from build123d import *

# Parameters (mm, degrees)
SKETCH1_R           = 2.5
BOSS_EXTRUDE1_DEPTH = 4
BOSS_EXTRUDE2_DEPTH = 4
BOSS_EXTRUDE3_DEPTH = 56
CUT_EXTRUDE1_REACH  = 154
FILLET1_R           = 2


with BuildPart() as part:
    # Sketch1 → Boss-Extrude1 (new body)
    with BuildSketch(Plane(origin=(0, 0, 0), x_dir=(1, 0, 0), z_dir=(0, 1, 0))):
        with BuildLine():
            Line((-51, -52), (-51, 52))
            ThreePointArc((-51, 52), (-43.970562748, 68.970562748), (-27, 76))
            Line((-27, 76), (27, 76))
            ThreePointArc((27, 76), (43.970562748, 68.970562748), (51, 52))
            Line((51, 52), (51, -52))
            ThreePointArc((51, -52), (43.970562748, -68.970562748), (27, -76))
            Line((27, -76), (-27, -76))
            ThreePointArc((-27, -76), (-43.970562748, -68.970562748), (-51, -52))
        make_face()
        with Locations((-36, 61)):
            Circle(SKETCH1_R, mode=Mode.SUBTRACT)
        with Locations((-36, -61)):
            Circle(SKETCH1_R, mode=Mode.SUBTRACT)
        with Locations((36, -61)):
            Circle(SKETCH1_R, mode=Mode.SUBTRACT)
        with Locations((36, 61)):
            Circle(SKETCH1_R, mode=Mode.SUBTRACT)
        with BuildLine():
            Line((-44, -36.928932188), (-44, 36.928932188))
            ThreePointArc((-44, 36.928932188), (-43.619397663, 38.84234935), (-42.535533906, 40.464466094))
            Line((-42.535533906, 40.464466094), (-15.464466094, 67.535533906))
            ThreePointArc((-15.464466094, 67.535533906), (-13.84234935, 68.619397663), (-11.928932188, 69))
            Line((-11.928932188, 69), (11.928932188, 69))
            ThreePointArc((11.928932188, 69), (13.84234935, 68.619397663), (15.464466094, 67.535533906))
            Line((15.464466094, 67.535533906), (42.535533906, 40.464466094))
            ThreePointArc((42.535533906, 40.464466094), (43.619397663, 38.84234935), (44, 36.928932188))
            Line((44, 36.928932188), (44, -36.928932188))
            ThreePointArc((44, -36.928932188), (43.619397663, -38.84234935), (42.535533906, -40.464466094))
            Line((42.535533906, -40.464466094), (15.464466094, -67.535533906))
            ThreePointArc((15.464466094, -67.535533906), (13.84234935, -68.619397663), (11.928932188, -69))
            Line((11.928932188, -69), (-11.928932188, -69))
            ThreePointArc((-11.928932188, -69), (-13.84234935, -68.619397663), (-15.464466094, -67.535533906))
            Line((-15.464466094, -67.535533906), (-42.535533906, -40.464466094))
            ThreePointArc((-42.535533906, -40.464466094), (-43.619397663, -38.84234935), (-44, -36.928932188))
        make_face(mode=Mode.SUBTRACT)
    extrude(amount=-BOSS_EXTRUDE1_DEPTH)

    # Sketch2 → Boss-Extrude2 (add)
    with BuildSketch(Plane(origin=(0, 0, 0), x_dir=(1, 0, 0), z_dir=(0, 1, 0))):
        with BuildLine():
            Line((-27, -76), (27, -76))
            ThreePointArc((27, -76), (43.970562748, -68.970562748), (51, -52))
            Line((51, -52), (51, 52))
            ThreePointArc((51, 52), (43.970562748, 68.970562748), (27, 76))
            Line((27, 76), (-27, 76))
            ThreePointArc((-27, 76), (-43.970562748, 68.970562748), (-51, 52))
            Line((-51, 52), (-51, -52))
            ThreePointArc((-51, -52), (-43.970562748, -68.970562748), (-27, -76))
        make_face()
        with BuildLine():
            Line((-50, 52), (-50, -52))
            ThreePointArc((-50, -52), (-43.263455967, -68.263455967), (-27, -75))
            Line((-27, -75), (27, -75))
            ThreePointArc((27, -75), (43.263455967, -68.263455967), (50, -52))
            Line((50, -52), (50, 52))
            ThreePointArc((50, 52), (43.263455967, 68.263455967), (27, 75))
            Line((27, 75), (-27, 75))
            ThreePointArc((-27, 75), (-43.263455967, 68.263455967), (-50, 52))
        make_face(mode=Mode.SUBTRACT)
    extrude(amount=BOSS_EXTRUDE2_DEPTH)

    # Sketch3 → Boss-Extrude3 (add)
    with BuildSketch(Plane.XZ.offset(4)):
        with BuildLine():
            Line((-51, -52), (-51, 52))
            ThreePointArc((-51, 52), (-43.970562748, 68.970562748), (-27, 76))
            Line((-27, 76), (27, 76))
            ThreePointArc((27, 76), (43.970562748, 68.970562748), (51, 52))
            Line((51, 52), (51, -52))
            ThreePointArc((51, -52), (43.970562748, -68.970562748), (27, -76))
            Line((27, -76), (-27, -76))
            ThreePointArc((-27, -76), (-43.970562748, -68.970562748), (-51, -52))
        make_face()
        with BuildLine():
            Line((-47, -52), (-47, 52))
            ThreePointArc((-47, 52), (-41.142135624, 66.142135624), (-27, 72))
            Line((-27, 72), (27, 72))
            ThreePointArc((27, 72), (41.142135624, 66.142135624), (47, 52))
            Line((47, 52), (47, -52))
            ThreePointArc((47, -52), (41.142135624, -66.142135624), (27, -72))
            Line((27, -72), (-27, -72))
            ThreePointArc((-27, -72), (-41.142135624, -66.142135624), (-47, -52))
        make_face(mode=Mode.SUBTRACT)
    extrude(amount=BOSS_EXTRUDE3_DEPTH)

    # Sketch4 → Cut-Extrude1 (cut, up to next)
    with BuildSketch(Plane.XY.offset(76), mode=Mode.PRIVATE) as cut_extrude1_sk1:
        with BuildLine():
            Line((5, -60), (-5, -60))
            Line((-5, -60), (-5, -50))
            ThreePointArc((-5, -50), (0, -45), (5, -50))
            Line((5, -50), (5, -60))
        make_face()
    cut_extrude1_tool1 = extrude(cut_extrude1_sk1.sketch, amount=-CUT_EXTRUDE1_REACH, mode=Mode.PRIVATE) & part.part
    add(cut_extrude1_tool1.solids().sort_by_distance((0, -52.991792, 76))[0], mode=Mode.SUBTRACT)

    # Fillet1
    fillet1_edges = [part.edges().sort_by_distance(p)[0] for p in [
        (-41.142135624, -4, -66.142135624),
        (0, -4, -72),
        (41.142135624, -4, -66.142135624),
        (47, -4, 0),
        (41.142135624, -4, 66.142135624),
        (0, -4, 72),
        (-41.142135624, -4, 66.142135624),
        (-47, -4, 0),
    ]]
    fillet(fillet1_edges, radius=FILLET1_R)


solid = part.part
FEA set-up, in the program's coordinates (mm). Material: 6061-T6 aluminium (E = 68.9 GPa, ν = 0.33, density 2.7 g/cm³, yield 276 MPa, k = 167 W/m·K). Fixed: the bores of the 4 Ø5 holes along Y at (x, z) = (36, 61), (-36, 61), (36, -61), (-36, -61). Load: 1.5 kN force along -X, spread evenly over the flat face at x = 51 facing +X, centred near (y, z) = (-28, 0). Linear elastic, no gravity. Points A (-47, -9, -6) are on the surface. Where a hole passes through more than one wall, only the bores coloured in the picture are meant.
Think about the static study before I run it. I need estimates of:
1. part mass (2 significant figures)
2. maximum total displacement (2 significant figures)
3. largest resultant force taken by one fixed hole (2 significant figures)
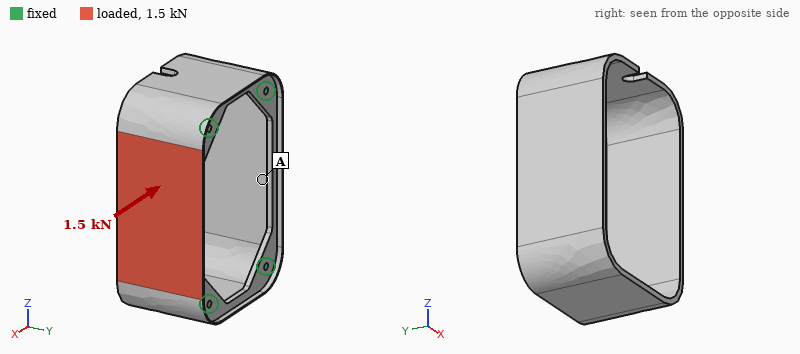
330 g
0.69 mm
1.2 kN
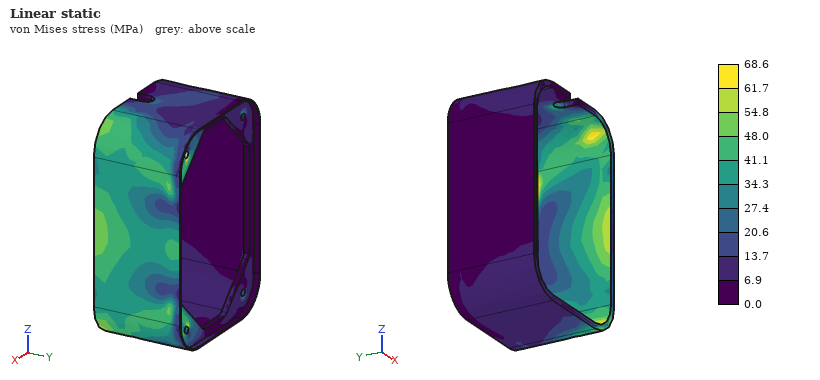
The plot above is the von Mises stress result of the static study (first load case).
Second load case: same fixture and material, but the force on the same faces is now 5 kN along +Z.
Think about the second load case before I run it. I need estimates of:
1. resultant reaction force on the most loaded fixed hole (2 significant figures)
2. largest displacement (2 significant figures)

2.8 kN
76 µm
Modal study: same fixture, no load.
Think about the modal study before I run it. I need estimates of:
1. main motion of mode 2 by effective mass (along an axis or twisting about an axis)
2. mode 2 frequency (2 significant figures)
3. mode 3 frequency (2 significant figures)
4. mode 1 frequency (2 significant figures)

along X
1200 Hz
1900 Hz
1000 Hz
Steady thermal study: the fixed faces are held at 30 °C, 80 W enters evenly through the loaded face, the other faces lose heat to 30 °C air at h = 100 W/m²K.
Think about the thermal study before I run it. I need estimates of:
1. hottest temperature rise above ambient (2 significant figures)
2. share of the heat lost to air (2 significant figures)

35 K
54 %
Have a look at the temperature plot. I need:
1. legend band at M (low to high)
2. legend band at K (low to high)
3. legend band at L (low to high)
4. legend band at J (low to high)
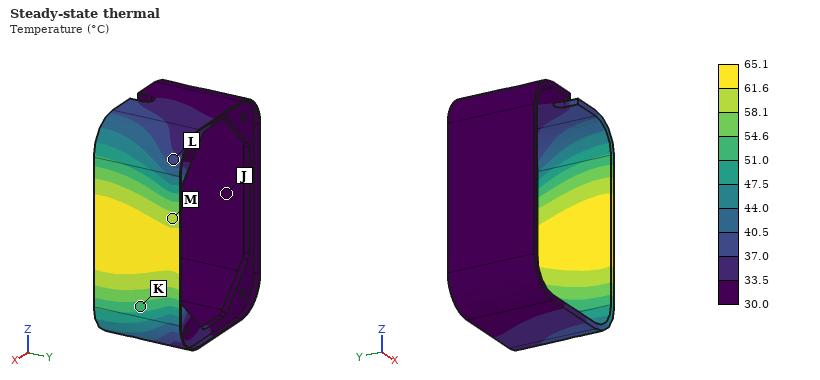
58.1 to 61.6 °C
51.0 to 54.6 °C
37.0 to 40.5 °C
30.0 to 33.5 °C
